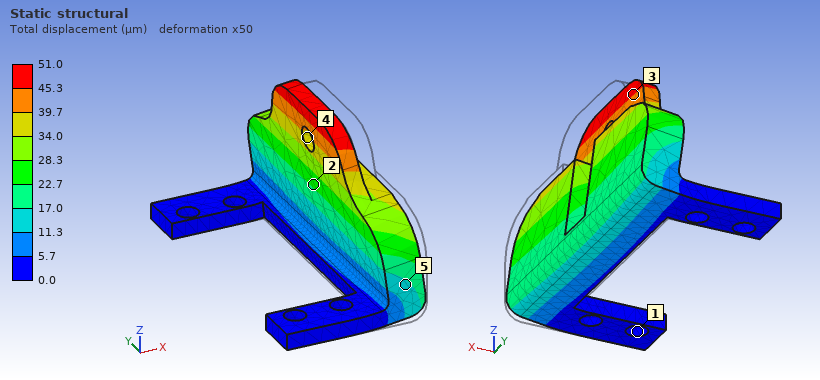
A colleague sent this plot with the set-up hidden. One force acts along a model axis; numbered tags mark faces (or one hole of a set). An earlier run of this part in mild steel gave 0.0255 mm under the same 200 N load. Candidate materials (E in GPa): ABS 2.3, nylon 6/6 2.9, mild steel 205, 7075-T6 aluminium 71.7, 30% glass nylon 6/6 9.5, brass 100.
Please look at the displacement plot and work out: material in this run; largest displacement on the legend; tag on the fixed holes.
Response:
brass
51.0 µm
1
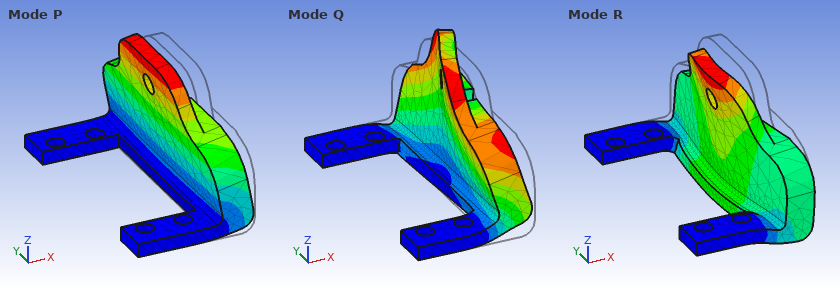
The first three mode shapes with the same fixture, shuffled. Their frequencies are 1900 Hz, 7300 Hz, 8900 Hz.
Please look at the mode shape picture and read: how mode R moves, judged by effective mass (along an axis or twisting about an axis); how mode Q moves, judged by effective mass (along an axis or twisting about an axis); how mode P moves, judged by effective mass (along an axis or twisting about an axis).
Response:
along Z
along Y
along X
